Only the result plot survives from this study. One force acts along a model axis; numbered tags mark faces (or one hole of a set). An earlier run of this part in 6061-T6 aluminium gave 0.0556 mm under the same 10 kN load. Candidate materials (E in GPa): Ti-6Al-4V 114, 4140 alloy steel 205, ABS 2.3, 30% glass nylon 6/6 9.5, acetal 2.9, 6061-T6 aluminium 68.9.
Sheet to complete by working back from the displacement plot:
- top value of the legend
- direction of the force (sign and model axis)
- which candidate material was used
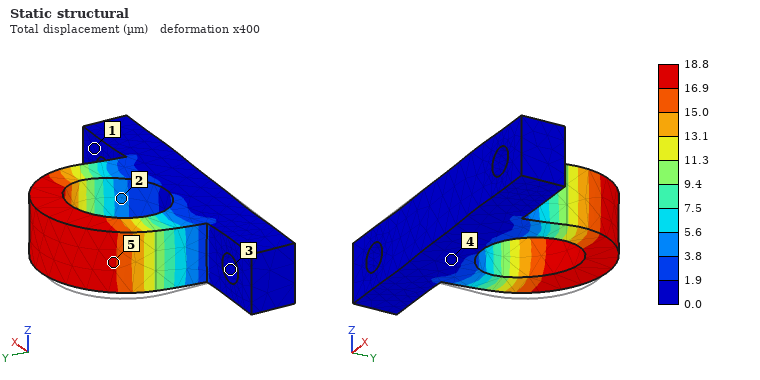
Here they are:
18.8 µm
+X
4140 alloy steel
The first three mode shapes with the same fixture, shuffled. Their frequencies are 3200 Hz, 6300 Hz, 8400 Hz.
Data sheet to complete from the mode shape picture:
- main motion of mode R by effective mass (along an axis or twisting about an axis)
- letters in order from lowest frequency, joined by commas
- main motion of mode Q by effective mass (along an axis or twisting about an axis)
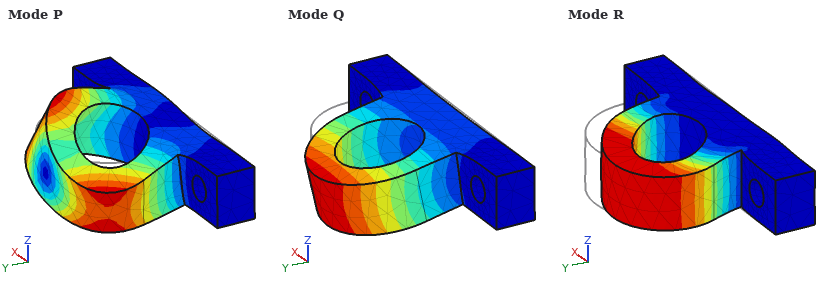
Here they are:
along X
Q, R, P
along Z
